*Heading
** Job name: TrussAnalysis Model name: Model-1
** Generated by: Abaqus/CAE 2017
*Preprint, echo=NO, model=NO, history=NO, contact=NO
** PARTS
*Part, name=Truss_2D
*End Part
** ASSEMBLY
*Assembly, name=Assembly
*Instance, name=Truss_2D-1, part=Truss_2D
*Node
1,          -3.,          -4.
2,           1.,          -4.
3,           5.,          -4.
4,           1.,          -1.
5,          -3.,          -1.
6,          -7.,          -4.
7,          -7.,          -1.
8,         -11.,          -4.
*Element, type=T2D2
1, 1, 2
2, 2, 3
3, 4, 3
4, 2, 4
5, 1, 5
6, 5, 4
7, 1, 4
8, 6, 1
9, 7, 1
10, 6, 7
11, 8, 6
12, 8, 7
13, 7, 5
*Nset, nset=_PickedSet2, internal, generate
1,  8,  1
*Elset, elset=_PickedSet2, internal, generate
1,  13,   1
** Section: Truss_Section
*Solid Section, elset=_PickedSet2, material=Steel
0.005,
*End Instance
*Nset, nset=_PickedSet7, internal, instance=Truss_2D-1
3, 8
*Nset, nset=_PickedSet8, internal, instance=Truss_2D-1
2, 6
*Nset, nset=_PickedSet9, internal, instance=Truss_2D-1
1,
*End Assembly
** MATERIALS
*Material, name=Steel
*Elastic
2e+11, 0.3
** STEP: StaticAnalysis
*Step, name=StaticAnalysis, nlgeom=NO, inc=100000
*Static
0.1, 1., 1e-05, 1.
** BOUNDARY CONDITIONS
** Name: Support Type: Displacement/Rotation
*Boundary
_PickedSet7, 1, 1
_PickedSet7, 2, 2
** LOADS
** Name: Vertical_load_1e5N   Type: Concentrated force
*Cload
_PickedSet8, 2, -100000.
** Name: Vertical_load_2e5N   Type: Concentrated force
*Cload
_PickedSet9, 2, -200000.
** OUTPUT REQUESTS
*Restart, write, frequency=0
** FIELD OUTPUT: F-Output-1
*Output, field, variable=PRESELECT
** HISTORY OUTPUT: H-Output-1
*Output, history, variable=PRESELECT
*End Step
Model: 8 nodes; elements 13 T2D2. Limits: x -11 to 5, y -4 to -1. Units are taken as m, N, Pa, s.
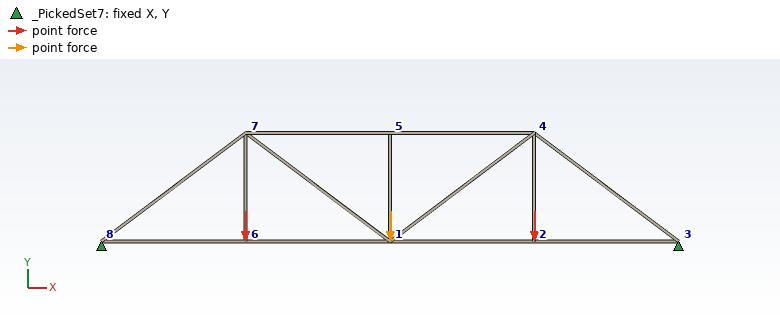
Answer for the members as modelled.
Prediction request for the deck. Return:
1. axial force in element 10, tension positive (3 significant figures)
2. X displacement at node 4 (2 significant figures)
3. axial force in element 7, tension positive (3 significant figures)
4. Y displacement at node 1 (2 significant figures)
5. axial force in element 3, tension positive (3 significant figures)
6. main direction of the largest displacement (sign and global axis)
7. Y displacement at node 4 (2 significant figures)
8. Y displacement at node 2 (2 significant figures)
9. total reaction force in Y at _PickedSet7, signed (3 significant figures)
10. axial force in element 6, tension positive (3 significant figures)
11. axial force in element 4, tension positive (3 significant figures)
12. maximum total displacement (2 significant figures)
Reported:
100000 N
-0.0016 m
1.67e+05 N
-0.0084 m
-3.33e+05 N
-Y
-0.0049 m
-0.0052 m
4.00e+05 N
-4.00e+05 N
1.00e+05 N
0.0084 m
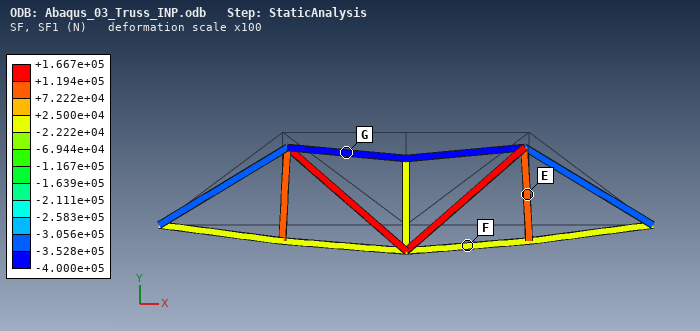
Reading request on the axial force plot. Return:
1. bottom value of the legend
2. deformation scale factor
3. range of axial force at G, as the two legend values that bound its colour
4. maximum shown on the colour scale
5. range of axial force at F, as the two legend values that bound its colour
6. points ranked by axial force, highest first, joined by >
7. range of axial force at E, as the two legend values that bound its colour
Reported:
-4.000e+05 N
100
-4.000e+05 to -3.528e+05 N
+1.667e+05 N
-2.222e+04 to +2.500e+04 N
E > F > G
+7.222e+04 to +1.194e+05 N
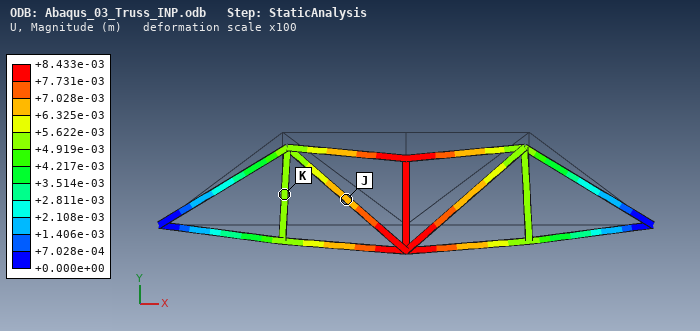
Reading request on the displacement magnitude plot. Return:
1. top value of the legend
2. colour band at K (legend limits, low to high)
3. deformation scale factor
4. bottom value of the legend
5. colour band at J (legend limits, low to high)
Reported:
+8.433e-03 m
+4.919e-03 to +5.622e-03 m
100
+0.000e+00 m
+6.325e-03 to +7.028e-03 m
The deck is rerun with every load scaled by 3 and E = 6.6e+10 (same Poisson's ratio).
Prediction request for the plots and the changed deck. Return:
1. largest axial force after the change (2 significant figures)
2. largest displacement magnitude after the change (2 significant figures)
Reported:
5.0e+05 N
0.077 m
